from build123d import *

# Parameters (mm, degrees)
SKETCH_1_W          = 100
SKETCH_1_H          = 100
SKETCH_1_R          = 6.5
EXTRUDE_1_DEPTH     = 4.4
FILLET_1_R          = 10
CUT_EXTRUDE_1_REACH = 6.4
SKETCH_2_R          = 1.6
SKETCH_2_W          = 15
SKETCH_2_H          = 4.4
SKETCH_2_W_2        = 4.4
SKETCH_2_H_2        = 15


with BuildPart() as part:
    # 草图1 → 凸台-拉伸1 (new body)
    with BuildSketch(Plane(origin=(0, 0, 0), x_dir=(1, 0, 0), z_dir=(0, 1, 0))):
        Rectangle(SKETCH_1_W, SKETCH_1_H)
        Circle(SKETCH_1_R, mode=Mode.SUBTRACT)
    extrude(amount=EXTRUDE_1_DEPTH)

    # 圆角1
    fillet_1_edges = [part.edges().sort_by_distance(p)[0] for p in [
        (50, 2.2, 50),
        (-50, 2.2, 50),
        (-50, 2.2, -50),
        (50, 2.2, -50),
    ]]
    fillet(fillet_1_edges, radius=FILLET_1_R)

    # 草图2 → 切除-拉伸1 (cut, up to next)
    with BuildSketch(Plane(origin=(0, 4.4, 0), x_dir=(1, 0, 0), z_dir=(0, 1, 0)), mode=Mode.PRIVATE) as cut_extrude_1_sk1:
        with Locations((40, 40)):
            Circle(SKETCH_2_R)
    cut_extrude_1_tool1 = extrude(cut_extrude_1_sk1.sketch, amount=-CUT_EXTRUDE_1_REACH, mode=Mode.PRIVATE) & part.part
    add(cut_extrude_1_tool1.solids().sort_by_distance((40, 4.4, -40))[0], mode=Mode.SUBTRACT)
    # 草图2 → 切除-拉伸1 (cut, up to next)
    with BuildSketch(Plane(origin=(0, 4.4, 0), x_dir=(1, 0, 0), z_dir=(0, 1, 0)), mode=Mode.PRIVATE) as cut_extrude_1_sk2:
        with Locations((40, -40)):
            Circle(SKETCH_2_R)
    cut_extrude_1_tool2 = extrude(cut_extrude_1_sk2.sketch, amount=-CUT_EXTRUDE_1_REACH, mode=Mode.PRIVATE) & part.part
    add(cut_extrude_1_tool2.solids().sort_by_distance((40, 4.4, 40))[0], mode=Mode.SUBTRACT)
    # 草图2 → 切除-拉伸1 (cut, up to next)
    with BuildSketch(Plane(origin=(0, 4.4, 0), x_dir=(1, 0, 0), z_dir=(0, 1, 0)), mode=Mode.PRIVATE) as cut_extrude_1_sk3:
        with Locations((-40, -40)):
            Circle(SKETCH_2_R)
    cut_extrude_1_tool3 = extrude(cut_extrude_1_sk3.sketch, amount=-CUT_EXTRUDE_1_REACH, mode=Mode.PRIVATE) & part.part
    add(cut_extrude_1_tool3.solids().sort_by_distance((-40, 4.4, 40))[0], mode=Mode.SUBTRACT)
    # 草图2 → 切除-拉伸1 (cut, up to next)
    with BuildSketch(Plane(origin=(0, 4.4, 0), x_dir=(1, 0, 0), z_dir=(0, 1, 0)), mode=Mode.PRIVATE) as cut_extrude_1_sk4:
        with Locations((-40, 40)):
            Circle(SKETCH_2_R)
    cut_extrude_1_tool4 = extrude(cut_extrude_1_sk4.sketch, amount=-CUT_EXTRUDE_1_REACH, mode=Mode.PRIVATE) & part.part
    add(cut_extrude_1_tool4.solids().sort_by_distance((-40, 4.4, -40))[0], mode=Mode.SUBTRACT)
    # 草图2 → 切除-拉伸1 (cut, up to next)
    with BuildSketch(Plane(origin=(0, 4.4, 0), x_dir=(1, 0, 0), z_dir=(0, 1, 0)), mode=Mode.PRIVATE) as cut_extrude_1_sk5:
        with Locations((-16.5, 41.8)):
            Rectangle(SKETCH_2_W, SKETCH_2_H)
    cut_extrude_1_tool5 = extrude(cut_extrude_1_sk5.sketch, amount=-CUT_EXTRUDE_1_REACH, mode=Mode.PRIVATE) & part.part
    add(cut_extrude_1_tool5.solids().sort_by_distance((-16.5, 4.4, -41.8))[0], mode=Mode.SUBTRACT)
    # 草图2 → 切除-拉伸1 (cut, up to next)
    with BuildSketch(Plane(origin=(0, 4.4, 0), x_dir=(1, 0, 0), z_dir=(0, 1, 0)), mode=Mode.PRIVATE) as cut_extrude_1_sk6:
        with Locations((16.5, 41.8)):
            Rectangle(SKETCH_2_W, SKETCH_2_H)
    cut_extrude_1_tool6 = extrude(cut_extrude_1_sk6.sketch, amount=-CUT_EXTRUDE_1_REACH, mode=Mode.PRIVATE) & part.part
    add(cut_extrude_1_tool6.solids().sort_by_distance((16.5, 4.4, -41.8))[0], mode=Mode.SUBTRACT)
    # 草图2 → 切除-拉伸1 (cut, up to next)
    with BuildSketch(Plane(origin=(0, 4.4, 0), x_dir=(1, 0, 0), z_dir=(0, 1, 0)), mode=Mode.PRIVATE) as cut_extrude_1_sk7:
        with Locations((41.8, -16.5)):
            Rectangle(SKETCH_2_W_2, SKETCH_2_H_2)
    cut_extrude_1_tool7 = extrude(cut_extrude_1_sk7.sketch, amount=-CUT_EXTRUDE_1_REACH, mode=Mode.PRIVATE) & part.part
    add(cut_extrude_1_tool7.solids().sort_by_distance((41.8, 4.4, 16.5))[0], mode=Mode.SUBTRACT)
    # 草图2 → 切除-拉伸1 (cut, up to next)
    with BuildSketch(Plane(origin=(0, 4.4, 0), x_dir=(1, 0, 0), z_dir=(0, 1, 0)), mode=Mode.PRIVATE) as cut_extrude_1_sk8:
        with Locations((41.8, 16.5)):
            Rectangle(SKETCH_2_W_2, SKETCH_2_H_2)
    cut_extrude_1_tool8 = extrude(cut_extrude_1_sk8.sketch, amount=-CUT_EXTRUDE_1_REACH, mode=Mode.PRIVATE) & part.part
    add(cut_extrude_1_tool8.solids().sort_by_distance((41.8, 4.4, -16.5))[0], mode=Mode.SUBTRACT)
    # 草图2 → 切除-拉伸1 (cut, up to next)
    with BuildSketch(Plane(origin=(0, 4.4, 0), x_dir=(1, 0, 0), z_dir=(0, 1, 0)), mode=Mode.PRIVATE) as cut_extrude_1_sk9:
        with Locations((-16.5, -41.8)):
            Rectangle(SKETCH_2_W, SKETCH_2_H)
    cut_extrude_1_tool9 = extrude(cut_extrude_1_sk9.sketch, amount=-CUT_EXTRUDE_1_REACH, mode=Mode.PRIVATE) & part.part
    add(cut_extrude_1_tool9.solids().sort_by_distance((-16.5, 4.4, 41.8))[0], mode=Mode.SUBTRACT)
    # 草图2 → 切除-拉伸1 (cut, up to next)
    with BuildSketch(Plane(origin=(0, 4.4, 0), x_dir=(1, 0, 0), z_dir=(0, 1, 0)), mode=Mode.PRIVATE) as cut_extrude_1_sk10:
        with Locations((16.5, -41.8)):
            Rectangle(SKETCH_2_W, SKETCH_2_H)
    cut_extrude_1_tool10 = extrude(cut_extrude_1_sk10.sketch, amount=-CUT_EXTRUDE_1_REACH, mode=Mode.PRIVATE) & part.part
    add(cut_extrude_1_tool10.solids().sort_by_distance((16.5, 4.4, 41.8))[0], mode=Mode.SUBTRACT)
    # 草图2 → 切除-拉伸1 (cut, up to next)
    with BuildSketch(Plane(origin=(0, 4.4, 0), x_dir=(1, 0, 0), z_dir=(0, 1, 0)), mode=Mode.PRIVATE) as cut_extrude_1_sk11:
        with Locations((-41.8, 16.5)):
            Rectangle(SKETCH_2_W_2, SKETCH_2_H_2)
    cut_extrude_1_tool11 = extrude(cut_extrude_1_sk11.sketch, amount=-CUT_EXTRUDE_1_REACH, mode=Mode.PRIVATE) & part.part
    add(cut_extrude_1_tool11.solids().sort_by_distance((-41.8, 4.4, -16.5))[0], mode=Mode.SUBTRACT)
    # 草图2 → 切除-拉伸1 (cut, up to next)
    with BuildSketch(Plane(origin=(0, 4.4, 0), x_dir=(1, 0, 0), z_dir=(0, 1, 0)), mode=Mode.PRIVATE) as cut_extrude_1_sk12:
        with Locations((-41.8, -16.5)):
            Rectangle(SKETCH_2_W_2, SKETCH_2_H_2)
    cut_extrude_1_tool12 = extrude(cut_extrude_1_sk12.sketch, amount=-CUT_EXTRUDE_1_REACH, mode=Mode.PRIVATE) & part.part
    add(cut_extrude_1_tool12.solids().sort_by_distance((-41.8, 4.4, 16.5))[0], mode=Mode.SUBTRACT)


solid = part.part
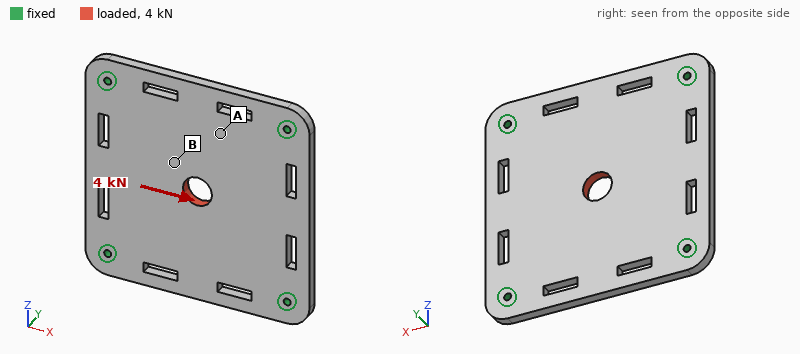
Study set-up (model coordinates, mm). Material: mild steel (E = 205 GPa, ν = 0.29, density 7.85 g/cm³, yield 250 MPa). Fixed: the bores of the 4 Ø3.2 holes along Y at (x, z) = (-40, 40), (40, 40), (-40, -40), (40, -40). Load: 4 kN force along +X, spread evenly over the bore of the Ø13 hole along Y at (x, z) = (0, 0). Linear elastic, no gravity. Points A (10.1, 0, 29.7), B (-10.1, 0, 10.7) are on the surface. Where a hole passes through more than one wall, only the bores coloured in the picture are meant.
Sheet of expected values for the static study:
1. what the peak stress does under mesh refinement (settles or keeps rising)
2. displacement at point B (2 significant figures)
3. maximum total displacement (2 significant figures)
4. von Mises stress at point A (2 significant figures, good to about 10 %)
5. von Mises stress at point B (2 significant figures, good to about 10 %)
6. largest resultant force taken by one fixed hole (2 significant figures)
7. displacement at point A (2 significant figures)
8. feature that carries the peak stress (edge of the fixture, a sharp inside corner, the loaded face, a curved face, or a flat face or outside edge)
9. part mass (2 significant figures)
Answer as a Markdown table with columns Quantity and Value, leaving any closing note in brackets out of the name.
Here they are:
| Quantity | Value |
|---|---|
| what the peak stress does under mesh refinement | keeps rising |
| displacement at point B | 3.3 µm |
| maximum total displacement | 4.5 µm |
| von Mises stress at point A | 8.1 MPa |
| von Mises stress at point B | 14 MPa |
| largest resultant force taken by one fixed hole | 1.1 kN |
| displacement at point A | 1.8 µm |
| feature that carries the peak stress | edge of the fixture |
| part mass | 320 g |
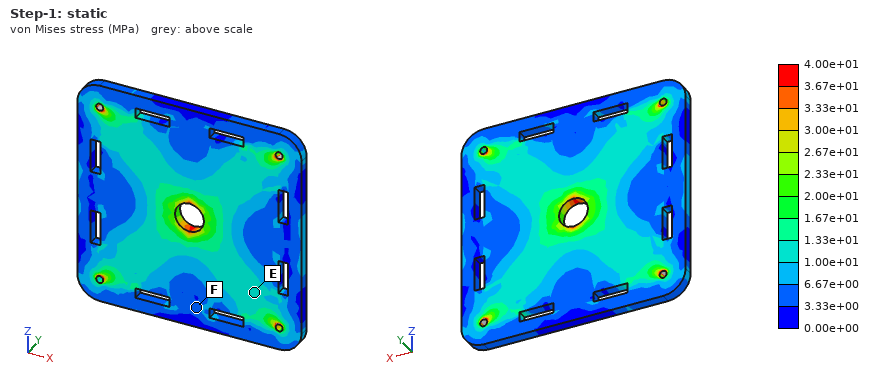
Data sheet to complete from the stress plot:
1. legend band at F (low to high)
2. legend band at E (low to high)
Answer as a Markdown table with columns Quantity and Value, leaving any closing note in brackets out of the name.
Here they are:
| Quantity | Value |
|---|---|
| legend band at F | 3.33e+00 to 6.67e+00 MPa |
| legend band at E | 1.00e+01 to 1.33e+01 MPa |
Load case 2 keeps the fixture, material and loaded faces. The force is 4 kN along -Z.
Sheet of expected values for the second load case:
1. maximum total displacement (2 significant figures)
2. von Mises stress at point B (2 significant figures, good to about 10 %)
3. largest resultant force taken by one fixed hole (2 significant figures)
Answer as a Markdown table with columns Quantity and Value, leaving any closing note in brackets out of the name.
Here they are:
| Quantity | Value |
|---|---|
| maximum total displacement | 4.5 µm |
| von Mises stress at point B | 15 MPa |
| largest resultant force taken by one fixed hole | 1.1 kN |
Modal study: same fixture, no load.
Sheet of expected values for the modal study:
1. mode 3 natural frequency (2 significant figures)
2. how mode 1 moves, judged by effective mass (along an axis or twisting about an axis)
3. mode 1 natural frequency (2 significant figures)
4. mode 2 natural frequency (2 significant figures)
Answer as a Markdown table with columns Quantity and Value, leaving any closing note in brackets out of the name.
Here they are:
| Quantity | Value |
|---|---|
| mode 3 natural frequency | 3700 Hz |
| how mode 1 moves, judged by effective mass | along Y |
| mode 1 natural frequency | 2200 Hz |
| mode 2 natural frequency | 3700 Hz |
